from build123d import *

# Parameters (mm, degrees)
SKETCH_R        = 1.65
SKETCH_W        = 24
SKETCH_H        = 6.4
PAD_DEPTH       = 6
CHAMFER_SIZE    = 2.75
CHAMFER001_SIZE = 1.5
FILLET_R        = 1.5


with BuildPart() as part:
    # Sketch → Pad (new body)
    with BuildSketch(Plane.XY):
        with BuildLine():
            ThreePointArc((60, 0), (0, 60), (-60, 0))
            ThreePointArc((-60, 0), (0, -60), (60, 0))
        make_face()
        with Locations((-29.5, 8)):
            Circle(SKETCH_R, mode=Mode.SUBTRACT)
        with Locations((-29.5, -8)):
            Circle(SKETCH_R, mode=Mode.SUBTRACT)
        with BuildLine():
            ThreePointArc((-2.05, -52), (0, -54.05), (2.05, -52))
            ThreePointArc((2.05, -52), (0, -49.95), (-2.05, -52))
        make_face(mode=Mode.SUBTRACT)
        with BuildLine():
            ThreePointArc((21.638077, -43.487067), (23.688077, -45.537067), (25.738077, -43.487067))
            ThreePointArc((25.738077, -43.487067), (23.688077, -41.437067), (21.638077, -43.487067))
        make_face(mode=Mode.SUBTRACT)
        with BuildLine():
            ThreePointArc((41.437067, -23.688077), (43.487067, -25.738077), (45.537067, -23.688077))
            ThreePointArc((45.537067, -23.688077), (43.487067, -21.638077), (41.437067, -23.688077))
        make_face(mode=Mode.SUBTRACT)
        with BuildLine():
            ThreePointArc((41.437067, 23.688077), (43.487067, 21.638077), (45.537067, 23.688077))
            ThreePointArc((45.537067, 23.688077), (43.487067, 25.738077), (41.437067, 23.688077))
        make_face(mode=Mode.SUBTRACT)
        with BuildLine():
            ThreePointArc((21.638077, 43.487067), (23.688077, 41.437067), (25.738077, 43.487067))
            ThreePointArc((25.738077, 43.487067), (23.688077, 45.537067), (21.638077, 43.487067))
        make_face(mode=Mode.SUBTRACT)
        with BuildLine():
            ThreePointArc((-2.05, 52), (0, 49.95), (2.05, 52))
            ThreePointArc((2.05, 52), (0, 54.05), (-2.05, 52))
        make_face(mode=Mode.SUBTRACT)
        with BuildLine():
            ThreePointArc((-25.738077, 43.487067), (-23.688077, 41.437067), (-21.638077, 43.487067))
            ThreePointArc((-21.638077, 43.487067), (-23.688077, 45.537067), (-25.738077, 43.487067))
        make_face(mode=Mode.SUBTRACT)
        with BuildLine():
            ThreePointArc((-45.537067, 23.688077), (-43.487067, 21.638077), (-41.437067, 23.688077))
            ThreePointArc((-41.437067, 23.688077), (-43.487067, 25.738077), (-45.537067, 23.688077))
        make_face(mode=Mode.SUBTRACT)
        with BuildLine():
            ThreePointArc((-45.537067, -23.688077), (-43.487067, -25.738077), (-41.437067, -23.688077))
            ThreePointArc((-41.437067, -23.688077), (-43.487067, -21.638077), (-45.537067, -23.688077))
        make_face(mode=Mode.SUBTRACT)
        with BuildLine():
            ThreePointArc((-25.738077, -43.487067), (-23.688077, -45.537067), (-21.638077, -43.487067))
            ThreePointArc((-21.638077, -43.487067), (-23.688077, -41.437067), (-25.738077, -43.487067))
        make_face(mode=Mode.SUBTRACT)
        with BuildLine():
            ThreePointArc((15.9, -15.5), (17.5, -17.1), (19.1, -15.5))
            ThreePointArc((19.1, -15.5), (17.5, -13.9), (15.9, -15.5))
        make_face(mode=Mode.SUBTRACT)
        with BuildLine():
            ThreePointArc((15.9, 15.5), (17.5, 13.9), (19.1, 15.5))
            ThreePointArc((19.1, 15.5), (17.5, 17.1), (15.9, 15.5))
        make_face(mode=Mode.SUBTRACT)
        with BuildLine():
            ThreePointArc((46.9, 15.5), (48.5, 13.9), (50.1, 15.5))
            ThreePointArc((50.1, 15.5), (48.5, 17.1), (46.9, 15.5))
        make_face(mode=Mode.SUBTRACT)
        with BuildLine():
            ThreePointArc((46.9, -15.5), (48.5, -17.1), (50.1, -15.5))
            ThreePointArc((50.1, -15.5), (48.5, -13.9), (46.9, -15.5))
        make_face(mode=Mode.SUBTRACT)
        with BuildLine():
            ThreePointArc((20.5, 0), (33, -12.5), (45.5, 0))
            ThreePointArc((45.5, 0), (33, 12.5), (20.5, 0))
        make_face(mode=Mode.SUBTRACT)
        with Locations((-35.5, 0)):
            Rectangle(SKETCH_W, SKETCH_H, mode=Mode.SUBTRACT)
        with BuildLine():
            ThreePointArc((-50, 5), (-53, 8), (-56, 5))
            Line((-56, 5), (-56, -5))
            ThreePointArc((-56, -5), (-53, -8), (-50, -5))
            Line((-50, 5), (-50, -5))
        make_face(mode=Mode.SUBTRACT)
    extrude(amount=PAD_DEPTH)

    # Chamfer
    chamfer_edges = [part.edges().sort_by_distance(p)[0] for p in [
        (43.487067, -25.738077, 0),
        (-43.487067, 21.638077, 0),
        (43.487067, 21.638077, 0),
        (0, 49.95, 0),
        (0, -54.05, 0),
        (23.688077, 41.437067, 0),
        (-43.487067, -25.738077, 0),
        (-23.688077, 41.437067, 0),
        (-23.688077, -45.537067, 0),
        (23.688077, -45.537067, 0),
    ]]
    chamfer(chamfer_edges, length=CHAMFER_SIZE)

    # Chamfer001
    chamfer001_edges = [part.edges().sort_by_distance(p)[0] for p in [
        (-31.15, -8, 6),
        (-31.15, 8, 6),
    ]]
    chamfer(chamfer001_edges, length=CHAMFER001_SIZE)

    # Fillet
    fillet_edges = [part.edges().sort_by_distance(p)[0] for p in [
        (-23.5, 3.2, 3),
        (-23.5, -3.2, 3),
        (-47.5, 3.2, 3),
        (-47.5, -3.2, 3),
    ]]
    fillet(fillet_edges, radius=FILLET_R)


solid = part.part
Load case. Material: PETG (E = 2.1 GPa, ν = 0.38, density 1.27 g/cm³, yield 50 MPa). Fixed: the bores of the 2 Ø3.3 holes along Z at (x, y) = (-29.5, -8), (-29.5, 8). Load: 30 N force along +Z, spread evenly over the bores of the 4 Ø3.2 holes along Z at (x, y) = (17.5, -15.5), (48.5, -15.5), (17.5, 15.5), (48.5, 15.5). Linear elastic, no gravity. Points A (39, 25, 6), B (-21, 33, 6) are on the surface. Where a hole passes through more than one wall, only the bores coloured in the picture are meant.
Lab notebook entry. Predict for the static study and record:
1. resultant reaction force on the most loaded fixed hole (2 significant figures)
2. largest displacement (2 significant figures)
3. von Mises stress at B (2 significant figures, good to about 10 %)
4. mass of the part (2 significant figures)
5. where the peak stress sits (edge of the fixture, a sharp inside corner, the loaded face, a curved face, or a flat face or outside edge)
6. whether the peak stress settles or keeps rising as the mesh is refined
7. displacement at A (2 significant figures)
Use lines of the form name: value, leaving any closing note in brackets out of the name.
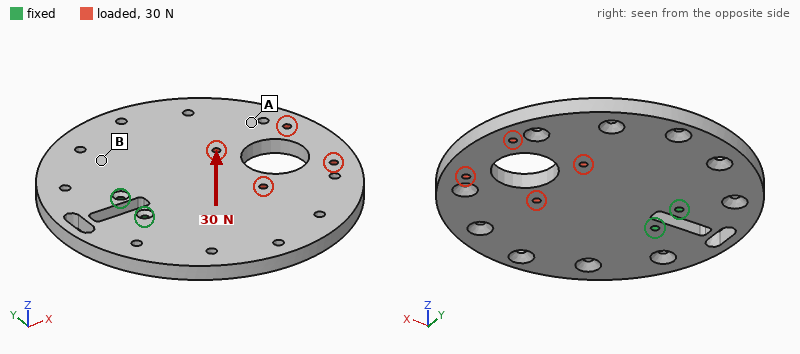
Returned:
resultant reaction force on the most loaded fixed hole: 15 N
largest displacement: 1.9 mm
von Mises stress at B: 1.9 MPa
mass of the part: 78 g
where the peak stress sits: edge of the fixture
whether the peak stress settles or keeps rising as the mesh is refined: keeps rising
displacement at A: 1.3 mm
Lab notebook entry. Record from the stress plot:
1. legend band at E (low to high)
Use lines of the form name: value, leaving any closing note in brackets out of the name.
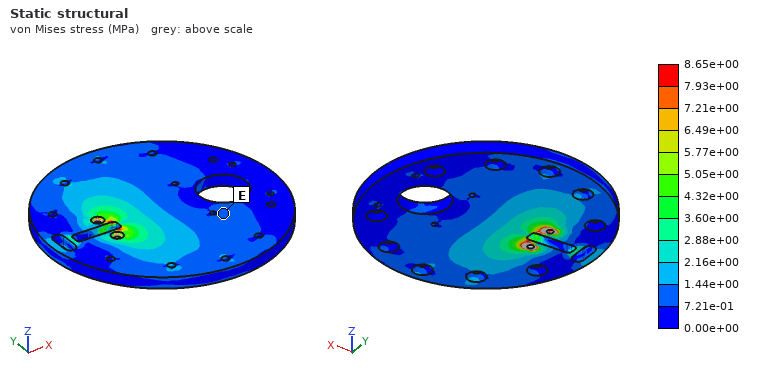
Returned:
legend band at E: 7.21e-01 to 1.44e+00 MPa
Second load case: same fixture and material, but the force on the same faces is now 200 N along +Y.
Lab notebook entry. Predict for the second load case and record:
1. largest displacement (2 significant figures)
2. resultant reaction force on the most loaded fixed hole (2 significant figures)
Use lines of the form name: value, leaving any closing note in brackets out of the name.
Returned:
largest displacement: 0.82 mm
resultant reaction force on the most loaded fixed hole: 630 N
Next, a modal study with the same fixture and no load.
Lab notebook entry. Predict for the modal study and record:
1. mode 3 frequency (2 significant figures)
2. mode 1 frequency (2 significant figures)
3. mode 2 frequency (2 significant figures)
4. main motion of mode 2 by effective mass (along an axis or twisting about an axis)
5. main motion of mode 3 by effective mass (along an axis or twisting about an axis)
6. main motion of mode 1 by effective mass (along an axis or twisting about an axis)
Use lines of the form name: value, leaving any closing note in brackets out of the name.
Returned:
mode 3 frequency: 420 Hz
mode 1 frequency: 140 Hz
mode 2 frequency: 250 Hz
main motion of mode 2 by effective mass: twisting about X
main motion of mode 3 by effective mass: along Y
main motion of mode 1 by effective mass: along Z
